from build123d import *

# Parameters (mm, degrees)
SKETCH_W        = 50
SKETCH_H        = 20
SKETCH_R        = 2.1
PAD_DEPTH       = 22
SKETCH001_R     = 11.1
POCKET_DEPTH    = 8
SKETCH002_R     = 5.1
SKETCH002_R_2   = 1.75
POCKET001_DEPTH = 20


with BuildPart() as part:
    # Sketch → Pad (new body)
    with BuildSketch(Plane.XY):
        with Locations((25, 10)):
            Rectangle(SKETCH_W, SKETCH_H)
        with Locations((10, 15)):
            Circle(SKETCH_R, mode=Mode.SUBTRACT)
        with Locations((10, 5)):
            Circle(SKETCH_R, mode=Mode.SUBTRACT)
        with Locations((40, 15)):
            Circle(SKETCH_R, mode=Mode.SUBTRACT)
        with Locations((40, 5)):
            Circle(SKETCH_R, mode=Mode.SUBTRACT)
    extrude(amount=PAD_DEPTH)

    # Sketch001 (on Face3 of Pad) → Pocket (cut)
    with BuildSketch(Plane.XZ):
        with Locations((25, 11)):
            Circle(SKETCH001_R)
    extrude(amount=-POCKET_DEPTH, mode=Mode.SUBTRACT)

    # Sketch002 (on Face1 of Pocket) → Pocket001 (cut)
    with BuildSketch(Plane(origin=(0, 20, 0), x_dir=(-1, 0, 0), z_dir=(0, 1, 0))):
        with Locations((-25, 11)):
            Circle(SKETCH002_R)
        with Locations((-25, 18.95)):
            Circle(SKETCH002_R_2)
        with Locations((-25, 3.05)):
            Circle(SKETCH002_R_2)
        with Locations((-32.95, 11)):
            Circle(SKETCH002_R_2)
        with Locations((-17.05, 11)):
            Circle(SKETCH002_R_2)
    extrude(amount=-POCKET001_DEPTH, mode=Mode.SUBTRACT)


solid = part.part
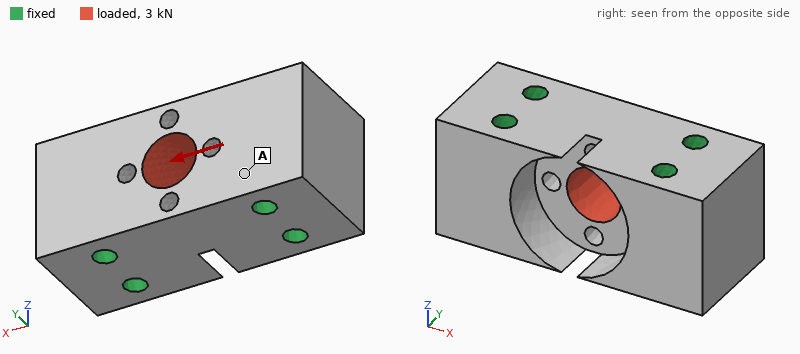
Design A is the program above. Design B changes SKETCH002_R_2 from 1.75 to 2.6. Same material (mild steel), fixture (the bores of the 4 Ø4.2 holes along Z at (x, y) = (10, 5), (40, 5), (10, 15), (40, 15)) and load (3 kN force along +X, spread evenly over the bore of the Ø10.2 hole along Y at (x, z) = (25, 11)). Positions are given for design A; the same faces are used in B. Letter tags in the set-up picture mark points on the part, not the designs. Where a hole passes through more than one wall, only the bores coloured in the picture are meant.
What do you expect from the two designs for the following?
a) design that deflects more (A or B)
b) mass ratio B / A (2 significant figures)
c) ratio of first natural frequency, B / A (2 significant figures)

B
0.97
0.95
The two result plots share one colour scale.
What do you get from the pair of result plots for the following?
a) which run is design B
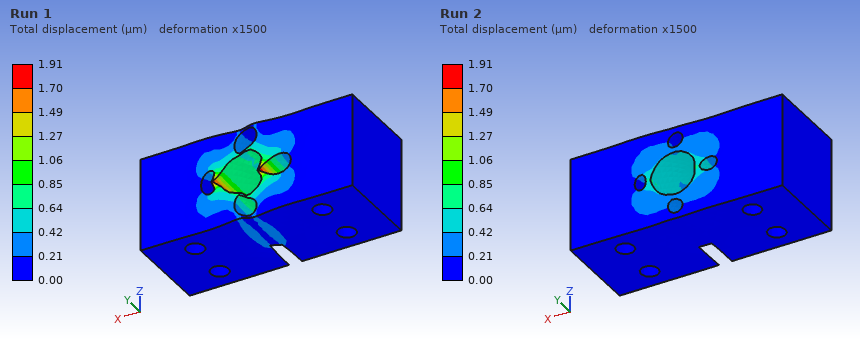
Run 1
